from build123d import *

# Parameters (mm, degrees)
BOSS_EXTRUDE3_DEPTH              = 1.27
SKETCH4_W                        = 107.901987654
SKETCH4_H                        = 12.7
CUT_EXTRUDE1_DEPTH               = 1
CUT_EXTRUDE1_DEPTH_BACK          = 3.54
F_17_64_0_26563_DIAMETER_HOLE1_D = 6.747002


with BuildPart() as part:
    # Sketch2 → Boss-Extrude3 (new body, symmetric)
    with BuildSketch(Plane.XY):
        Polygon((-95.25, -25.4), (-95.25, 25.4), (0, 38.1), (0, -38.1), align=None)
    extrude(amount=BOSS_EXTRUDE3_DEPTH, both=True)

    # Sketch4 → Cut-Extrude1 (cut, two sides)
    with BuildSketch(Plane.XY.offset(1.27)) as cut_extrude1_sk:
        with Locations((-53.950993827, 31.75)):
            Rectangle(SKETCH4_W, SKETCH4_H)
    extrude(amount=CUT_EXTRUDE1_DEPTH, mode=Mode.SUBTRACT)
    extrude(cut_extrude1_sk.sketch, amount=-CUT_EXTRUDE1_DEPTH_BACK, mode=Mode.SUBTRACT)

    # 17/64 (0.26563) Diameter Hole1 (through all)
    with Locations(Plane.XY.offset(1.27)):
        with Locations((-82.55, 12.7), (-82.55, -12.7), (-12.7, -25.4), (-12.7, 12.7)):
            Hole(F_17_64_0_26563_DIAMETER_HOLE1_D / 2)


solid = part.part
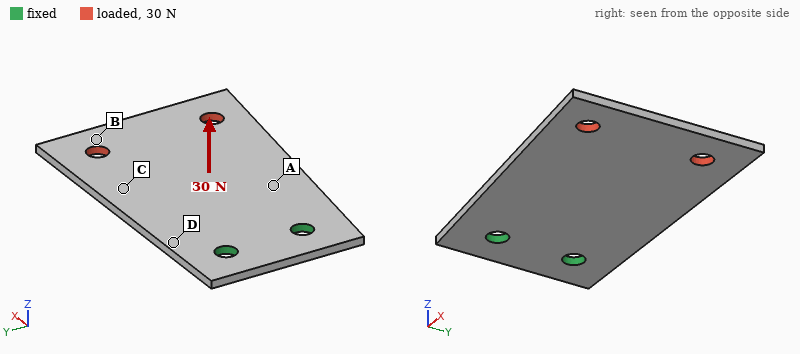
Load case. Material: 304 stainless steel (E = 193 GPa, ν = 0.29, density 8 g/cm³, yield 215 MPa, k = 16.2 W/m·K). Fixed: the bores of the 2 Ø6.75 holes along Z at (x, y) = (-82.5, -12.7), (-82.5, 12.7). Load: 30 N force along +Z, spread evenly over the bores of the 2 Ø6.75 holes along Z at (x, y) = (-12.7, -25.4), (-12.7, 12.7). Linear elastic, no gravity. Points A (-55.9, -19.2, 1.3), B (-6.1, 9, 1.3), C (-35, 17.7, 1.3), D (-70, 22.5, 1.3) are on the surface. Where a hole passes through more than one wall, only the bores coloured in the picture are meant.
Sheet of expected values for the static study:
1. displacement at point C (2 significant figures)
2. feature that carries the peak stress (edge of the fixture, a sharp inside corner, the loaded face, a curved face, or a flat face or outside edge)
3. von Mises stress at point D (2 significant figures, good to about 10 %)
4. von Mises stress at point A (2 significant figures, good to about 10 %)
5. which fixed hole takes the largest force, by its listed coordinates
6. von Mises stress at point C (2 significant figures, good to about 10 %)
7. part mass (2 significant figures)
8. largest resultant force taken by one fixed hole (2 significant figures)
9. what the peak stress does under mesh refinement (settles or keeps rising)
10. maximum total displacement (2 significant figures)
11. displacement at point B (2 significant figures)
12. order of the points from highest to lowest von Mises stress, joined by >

0.11 mm
edge of the fixture
28 MPa
20 MPa
(-82.5, -12.7)
11 MPa
110 g
21 N
keeps rising
0.28 mm
0.24 mm
D > A > C > B
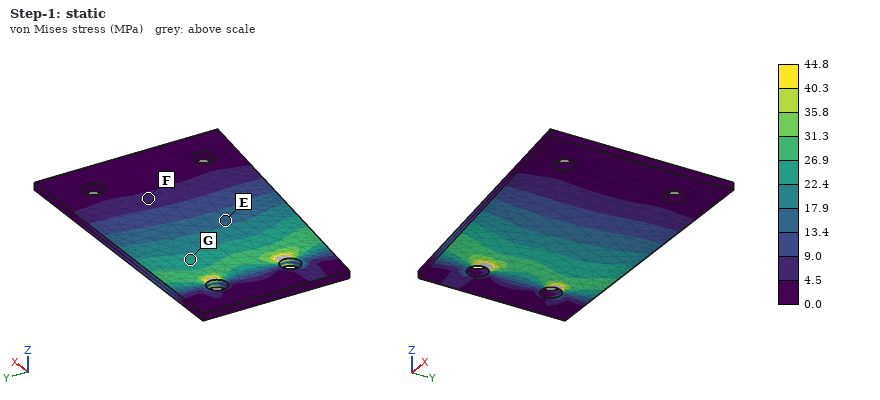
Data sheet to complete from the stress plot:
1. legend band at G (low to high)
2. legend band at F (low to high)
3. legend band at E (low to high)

22.4 to 26.9 MPa
4.5 to 9.0 MPa
13.4 to 17.9 MPa
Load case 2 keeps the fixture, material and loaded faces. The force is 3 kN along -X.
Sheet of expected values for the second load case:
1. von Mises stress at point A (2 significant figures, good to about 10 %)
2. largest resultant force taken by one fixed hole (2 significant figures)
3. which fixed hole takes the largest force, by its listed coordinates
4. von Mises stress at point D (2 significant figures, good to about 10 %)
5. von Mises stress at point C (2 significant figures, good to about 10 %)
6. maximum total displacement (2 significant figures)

27 MPa
2.1 kN
(-82.5, -12.7)
8.4 MPa
18 MPa
16 µm
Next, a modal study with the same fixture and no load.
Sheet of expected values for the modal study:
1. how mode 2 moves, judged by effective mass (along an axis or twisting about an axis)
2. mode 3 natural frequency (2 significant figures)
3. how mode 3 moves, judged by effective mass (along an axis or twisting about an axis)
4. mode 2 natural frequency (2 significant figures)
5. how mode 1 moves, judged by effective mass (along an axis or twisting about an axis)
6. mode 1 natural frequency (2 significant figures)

twisting about X
1900 Hz
along Z
890 Hz
along Z
300 Hz
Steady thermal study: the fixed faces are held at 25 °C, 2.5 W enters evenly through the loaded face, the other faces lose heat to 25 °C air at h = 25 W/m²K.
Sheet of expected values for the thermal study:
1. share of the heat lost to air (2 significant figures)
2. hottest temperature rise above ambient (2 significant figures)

90 %
24 K
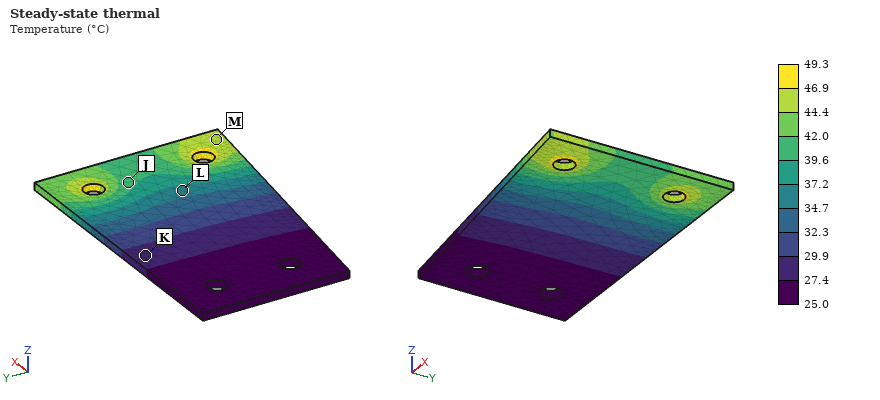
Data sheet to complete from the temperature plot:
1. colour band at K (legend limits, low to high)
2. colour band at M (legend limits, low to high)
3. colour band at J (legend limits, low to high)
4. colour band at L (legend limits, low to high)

27.4 to 29.9 °C
44.4 to 46.9 °C
39.6 to 42.0 °C
34.7 to 37.2 °C
